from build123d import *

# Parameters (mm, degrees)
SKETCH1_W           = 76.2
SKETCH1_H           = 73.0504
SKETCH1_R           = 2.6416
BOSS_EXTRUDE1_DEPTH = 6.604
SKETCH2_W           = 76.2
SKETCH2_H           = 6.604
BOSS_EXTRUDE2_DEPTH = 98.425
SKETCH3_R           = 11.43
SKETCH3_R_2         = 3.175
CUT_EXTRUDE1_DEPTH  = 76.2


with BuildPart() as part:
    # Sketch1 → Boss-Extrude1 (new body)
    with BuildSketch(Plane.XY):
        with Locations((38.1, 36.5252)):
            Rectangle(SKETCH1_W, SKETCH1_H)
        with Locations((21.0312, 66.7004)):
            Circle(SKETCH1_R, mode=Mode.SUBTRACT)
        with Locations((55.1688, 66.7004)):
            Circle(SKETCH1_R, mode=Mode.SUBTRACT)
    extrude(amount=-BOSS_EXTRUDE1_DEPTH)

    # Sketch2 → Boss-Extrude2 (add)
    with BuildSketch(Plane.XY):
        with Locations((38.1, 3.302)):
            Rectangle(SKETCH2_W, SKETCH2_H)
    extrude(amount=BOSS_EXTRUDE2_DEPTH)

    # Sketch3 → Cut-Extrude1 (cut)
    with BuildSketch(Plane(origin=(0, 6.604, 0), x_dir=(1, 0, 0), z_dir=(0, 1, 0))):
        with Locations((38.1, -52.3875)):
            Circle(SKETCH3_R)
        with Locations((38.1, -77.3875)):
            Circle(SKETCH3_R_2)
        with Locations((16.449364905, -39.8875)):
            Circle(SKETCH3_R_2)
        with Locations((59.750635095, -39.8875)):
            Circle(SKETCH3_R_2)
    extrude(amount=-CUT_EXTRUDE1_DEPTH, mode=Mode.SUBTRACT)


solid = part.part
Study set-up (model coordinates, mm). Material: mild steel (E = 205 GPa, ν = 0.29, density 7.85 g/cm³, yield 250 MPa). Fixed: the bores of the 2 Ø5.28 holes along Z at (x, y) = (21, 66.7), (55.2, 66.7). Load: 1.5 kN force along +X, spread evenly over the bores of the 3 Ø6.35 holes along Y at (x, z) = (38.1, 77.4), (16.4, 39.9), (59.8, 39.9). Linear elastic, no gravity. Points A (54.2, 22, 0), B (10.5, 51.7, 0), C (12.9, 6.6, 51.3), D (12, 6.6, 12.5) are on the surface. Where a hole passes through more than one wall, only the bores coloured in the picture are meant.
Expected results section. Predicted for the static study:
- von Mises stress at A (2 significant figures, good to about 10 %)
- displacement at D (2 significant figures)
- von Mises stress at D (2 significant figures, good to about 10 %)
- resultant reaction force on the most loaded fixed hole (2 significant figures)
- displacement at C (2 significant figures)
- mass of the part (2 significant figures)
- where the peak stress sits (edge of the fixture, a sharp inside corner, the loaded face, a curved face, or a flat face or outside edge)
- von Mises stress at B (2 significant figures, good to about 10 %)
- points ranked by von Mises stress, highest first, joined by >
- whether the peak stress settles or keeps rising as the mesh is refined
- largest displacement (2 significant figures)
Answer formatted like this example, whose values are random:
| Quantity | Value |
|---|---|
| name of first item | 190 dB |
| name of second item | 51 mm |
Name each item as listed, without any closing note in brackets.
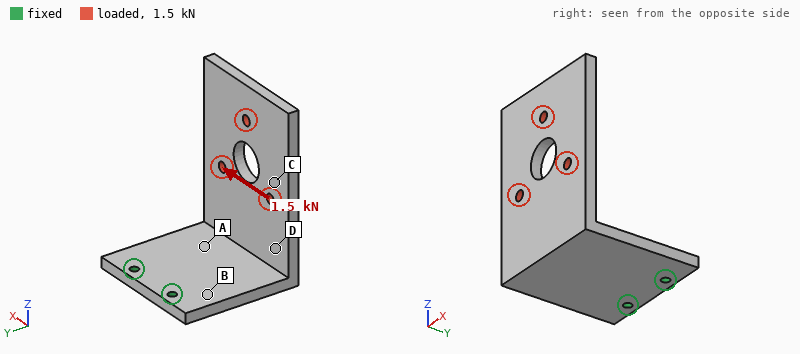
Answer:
| Quantity | Value |
|---|---|
| von Mises stress at A | 110 MPa |
| displacement at D | 0.20 mm |
| von Mises stress at D | 49 MPa |
| resultant reaction force on the most loaded fixed hole | 3.2 kN |
| displacement at C | 0.41 mm |
| mass of the part | 650 g |
| where the peak stress sits | edge of the fixture |
| von Mises stress at B | 75 MPa |
| points ranked by von Mises stress, highest first, joined by > | A > B > D > C |
| whether the peak stress settles or keeps rising as the mesh is refined | keeps rising |
| largest displacement | 0.72 mm |
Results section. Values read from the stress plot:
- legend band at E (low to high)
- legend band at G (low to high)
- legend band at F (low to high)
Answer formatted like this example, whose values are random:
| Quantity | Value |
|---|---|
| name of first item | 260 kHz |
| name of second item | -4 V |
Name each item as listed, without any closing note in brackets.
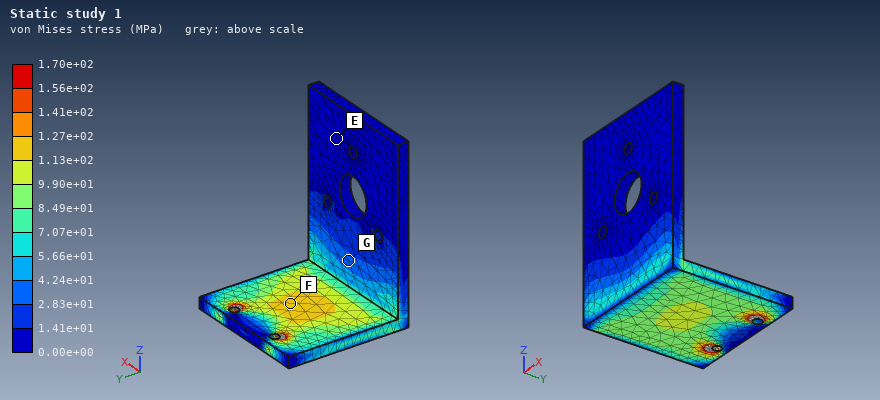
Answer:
| Quantity | Value |
|---|---|
| legend band at E | 0.00e+00 to 1.41e+01 MPa |
| legend band at G | 2.83e+01 to 4.24e+01 MPa |
| legend band at F | 1.13e+02 to 1.27e+02 MPa |
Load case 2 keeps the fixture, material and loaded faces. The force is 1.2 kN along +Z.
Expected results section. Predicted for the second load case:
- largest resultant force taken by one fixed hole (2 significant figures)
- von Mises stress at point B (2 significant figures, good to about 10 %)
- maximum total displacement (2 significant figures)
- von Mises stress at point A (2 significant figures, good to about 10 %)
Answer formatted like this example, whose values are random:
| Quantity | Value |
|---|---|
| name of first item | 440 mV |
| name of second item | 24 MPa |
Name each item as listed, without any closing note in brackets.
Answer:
| Quantity | Value |
|---|---|
| largest resultant force taken by one fixed hole | 600 N |
| von Mises stress at point B | 97 MPa |
| maximum total displacement | 0.77 mm |
| von Mises stress at point A | 37 MPa |
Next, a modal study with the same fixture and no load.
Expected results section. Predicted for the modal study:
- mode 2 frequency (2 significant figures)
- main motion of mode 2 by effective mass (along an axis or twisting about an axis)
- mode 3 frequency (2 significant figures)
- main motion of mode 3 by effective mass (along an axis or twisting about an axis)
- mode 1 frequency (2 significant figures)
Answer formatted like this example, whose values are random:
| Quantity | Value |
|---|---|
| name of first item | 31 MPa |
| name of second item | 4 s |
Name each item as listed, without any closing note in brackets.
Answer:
| Quantity | Value |
|---|---|
| mode 2 frequency | 460 Hz |
| main motion of mode 2 by effective mass | along X |
| mode 3 frequency | 770 Hz |
| main motion of mode 3 by effective mass | along Z |
| mode 1 frequency | 260 Hz |
